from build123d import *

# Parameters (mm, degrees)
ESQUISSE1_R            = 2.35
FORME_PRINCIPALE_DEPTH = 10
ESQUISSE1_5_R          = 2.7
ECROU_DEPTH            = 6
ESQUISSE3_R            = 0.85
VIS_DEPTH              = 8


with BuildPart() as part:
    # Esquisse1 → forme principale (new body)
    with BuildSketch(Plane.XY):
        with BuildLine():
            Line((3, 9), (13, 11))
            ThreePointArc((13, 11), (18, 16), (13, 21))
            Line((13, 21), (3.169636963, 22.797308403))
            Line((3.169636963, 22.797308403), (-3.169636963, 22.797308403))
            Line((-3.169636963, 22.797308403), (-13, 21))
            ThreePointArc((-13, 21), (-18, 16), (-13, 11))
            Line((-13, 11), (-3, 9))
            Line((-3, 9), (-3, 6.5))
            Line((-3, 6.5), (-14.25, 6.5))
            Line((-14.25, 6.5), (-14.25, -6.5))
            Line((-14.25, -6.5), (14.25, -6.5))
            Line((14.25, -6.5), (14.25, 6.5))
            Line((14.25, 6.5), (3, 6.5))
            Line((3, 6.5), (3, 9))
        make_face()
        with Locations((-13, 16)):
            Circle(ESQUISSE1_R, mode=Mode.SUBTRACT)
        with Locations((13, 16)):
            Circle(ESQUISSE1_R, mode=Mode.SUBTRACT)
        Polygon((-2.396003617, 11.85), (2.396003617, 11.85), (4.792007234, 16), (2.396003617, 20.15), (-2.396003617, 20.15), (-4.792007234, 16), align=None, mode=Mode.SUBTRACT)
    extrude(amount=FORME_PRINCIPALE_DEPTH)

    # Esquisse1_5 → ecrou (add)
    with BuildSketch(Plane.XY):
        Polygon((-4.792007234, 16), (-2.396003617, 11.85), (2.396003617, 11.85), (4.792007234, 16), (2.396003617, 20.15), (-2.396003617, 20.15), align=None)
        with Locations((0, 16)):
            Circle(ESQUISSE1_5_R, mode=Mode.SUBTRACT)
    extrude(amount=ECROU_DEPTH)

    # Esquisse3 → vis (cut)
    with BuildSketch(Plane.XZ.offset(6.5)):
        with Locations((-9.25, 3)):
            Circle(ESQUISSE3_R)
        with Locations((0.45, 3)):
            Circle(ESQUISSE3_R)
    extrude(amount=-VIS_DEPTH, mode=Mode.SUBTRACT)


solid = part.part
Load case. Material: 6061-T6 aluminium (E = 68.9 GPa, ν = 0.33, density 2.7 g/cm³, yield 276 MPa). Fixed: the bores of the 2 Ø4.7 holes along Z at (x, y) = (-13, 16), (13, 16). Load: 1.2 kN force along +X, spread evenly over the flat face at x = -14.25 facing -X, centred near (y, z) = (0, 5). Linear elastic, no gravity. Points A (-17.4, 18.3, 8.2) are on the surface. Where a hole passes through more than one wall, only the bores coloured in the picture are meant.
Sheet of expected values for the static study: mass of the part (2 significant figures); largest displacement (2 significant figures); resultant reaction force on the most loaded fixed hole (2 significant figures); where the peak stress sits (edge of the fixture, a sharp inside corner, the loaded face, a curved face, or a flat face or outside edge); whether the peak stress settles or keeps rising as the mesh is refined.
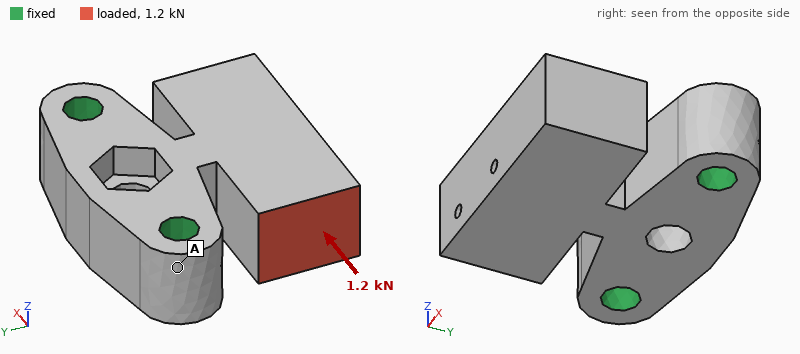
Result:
19 g
0.13 mm
1.1 kN
a sharp inside corner
keeps rising
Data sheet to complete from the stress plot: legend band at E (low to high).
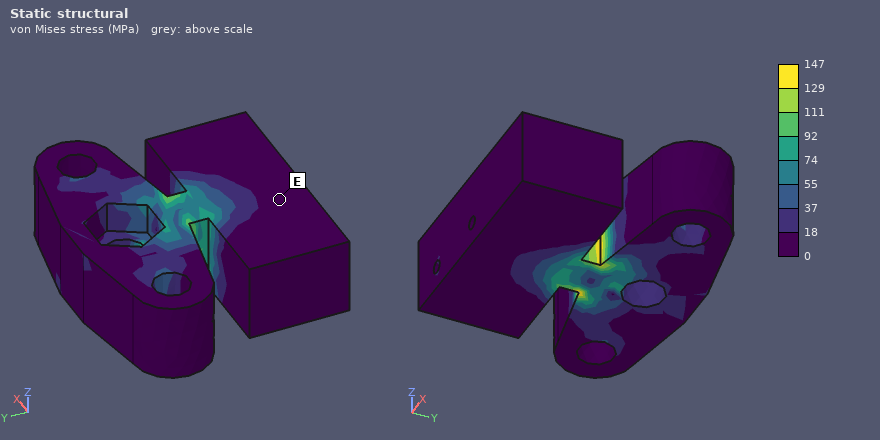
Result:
0 to 18 MPa
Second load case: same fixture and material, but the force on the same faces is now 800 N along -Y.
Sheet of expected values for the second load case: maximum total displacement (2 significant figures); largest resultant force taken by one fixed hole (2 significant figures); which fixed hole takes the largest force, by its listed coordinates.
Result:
0.15 mm
1.1 kN
(-13, 16)
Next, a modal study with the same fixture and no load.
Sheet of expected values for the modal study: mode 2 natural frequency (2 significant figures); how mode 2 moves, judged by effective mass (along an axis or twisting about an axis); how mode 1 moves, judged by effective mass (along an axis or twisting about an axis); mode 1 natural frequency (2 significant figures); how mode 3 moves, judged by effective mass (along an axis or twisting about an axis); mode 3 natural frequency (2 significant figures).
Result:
6100 Hz
along Z
along X
5300 Hz
twisting about Y
9100 Hz
